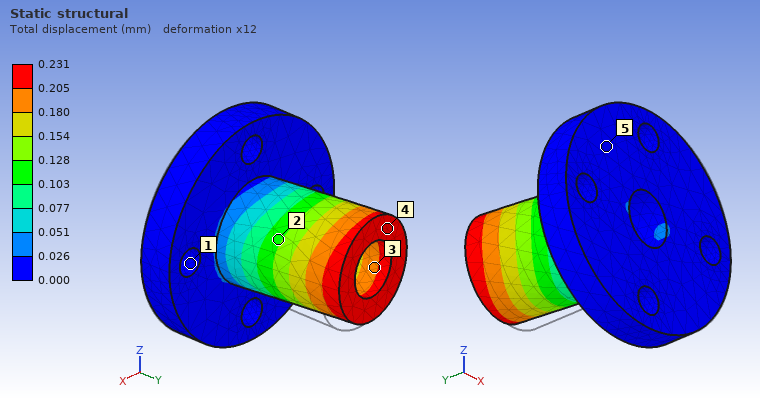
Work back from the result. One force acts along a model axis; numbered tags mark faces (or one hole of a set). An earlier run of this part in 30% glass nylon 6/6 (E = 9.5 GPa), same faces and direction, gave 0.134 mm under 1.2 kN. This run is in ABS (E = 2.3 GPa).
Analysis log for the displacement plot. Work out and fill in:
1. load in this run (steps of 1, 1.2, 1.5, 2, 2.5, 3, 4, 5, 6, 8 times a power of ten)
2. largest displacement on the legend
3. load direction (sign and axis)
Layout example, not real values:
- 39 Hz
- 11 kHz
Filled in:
- 500 N
- 0.231 mm
- -X
